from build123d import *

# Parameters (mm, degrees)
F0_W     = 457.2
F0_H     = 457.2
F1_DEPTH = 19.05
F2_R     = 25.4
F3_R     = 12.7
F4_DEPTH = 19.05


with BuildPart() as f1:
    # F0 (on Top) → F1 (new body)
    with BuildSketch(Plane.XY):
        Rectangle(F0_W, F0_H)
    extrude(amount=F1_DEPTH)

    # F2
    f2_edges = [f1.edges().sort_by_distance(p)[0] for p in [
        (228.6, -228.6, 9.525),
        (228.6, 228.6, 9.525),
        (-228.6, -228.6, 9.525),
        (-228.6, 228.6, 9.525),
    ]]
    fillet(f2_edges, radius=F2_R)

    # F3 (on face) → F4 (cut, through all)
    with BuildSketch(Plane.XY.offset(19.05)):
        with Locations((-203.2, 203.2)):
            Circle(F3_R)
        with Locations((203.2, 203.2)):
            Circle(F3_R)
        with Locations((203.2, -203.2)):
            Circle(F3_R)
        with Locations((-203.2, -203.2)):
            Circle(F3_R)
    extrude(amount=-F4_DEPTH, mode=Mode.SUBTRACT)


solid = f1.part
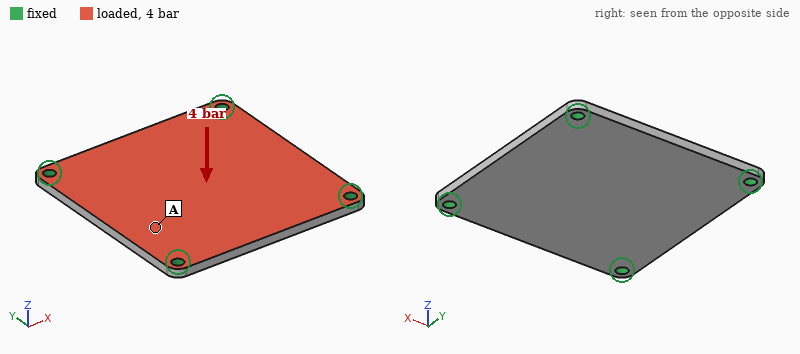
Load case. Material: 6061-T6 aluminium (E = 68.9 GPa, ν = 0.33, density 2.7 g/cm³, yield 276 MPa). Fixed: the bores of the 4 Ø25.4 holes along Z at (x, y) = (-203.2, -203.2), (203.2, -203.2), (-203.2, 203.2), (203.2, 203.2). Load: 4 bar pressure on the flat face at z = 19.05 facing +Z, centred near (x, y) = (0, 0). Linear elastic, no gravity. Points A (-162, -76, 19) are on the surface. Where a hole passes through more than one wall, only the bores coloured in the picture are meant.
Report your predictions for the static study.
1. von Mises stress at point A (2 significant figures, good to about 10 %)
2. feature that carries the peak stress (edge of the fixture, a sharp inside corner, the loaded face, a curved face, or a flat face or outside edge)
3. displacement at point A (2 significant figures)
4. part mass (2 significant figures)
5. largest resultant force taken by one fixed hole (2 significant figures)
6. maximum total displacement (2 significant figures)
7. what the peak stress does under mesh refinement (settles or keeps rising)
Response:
40 MPa
edge of the fixture
1.0 mm
11 kg
21 kN
1.9 mm
keeps rising
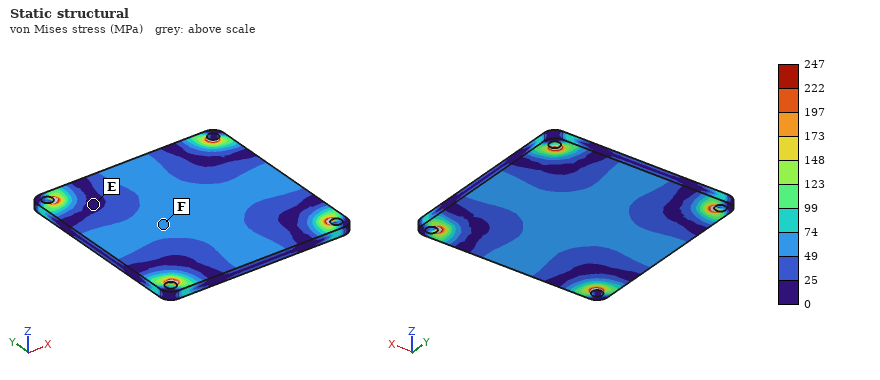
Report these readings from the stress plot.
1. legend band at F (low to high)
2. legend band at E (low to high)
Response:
49 to 74 MPa
0 to 25 MPa
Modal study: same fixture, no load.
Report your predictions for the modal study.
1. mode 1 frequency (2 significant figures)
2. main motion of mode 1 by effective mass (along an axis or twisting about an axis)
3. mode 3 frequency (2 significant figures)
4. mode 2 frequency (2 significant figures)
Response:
390 Hz
along Z
670 Hz
670 Hz
